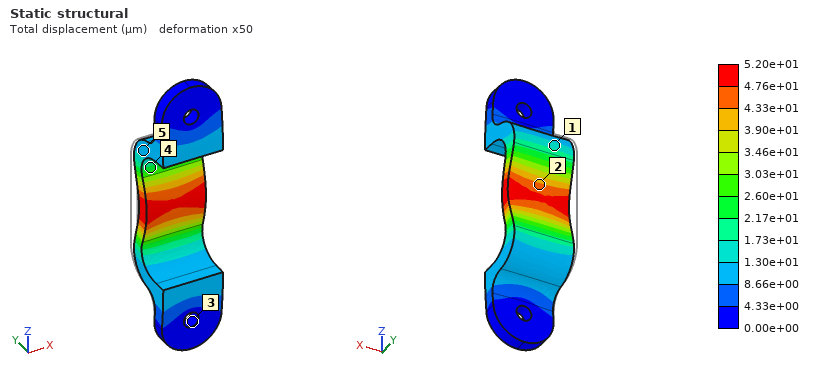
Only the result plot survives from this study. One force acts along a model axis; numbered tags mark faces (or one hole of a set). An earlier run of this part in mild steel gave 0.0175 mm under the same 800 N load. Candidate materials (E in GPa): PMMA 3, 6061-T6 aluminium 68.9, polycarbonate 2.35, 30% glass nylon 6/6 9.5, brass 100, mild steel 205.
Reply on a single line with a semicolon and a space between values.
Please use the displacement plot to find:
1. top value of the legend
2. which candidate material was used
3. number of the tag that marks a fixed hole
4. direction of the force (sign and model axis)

5.20e+01 µm; 6061-T6 aluminium; 3; -Y
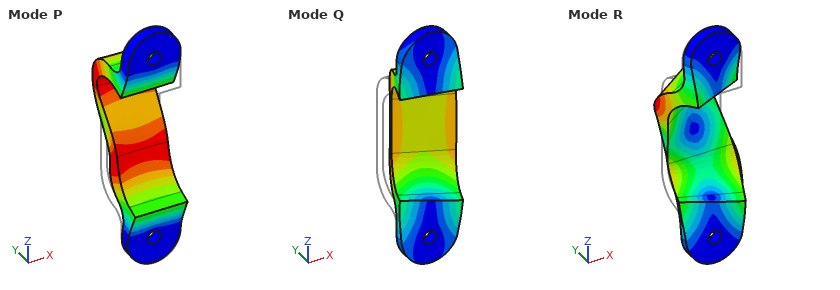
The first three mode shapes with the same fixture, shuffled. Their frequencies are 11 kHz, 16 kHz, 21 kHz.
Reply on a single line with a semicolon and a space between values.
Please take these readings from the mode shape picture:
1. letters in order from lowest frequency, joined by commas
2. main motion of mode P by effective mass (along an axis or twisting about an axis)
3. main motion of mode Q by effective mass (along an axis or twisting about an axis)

Q, P, R; along Z; along X
